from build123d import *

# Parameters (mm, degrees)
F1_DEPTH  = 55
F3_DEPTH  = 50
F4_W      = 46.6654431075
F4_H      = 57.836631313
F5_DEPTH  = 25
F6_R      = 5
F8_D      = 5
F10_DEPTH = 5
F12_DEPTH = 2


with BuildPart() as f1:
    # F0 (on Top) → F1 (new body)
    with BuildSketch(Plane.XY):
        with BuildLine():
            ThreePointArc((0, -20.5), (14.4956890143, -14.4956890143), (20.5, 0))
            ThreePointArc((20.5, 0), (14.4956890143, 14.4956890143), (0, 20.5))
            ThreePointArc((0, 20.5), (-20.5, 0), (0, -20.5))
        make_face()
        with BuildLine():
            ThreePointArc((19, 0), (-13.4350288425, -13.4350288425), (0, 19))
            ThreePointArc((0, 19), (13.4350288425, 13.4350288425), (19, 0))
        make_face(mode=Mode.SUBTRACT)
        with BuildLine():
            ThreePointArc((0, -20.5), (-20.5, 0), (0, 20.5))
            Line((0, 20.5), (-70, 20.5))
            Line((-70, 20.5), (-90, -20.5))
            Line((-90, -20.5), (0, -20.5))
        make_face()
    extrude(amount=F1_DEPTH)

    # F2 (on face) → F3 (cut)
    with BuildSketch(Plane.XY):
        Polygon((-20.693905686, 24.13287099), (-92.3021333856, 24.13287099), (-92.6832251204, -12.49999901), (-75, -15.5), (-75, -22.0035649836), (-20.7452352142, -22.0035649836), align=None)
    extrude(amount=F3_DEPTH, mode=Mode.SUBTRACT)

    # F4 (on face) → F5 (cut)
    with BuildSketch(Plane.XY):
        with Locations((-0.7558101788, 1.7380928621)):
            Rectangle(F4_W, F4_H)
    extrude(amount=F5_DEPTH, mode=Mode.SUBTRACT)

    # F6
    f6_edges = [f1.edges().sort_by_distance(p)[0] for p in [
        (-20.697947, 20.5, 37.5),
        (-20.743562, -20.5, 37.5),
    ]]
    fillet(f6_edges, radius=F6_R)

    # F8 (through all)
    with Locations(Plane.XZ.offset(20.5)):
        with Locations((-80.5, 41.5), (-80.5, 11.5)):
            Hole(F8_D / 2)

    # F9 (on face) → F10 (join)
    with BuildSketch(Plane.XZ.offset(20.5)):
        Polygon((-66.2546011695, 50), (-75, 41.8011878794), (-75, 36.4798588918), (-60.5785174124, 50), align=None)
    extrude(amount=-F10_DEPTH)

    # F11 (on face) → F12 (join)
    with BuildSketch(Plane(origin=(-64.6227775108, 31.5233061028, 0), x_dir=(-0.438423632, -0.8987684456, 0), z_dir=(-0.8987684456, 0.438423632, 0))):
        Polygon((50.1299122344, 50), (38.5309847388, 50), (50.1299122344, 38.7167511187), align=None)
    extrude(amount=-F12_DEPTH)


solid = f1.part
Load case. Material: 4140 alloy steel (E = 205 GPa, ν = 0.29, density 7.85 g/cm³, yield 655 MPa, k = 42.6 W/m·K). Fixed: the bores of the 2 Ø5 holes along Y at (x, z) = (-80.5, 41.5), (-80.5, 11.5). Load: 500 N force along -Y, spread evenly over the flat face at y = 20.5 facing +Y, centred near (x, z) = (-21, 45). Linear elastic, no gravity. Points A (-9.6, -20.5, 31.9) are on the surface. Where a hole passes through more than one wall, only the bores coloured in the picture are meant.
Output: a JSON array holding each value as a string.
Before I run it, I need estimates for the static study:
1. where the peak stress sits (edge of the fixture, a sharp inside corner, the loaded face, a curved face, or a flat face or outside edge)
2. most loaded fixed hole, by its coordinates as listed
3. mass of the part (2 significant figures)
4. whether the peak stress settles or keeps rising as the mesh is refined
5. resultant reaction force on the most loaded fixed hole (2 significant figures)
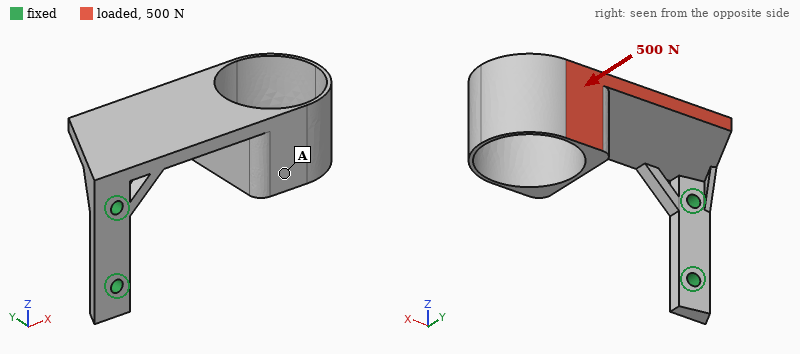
["edge of the fixture", "(-80.5, 41.5)", "220 g", "keeps rising", "510 N"]
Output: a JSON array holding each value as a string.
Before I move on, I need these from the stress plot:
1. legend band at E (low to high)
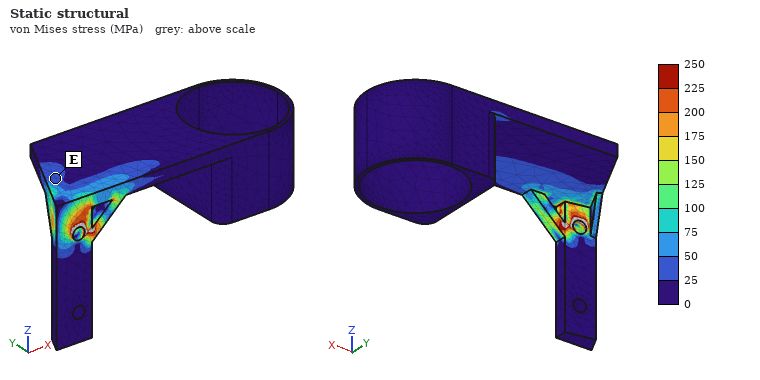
["25 to 50 MPa"]
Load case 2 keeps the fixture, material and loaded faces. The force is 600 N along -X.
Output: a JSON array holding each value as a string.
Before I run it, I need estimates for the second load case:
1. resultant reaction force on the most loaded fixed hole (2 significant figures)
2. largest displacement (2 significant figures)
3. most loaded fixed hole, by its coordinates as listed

["640 N", "0.44 mm", "(-80.5, 41.5)"]
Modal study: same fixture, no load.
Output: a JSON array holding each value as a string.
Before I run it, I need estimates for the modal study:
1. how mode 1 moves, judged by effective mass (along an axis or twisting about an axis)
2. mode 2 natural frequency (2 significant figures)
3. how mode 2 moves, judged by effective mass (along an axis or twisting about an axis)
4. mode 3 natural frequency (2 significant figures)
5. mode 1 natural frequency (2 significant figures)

["along Z", "530 Hz", "along Y", "1100 Hz", "370 Hz"]
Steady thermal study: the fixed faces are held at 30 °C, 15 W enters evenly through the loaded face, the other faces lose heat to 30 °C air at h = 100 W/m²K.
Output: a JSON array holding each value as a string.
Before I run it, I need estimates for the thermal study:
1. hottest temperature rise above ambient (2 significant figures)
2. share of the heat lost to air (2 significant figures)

["30 K", "93 %"]
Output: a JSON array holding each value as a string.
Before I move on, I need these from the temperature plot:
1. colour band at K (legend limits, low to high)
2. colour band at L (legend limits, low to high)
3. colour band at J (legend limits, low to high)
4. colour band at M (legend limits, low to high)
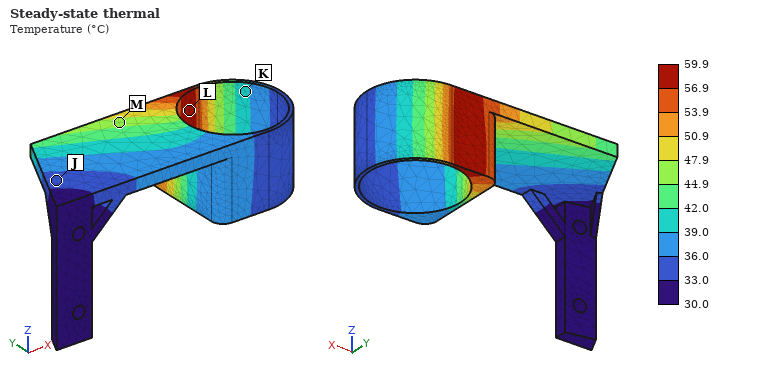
["39.0 to 42.0 °C", "56.9 to 59.9 °C", "33.0 to 36.0 °C", "44.9 to 47.9 °C"]
